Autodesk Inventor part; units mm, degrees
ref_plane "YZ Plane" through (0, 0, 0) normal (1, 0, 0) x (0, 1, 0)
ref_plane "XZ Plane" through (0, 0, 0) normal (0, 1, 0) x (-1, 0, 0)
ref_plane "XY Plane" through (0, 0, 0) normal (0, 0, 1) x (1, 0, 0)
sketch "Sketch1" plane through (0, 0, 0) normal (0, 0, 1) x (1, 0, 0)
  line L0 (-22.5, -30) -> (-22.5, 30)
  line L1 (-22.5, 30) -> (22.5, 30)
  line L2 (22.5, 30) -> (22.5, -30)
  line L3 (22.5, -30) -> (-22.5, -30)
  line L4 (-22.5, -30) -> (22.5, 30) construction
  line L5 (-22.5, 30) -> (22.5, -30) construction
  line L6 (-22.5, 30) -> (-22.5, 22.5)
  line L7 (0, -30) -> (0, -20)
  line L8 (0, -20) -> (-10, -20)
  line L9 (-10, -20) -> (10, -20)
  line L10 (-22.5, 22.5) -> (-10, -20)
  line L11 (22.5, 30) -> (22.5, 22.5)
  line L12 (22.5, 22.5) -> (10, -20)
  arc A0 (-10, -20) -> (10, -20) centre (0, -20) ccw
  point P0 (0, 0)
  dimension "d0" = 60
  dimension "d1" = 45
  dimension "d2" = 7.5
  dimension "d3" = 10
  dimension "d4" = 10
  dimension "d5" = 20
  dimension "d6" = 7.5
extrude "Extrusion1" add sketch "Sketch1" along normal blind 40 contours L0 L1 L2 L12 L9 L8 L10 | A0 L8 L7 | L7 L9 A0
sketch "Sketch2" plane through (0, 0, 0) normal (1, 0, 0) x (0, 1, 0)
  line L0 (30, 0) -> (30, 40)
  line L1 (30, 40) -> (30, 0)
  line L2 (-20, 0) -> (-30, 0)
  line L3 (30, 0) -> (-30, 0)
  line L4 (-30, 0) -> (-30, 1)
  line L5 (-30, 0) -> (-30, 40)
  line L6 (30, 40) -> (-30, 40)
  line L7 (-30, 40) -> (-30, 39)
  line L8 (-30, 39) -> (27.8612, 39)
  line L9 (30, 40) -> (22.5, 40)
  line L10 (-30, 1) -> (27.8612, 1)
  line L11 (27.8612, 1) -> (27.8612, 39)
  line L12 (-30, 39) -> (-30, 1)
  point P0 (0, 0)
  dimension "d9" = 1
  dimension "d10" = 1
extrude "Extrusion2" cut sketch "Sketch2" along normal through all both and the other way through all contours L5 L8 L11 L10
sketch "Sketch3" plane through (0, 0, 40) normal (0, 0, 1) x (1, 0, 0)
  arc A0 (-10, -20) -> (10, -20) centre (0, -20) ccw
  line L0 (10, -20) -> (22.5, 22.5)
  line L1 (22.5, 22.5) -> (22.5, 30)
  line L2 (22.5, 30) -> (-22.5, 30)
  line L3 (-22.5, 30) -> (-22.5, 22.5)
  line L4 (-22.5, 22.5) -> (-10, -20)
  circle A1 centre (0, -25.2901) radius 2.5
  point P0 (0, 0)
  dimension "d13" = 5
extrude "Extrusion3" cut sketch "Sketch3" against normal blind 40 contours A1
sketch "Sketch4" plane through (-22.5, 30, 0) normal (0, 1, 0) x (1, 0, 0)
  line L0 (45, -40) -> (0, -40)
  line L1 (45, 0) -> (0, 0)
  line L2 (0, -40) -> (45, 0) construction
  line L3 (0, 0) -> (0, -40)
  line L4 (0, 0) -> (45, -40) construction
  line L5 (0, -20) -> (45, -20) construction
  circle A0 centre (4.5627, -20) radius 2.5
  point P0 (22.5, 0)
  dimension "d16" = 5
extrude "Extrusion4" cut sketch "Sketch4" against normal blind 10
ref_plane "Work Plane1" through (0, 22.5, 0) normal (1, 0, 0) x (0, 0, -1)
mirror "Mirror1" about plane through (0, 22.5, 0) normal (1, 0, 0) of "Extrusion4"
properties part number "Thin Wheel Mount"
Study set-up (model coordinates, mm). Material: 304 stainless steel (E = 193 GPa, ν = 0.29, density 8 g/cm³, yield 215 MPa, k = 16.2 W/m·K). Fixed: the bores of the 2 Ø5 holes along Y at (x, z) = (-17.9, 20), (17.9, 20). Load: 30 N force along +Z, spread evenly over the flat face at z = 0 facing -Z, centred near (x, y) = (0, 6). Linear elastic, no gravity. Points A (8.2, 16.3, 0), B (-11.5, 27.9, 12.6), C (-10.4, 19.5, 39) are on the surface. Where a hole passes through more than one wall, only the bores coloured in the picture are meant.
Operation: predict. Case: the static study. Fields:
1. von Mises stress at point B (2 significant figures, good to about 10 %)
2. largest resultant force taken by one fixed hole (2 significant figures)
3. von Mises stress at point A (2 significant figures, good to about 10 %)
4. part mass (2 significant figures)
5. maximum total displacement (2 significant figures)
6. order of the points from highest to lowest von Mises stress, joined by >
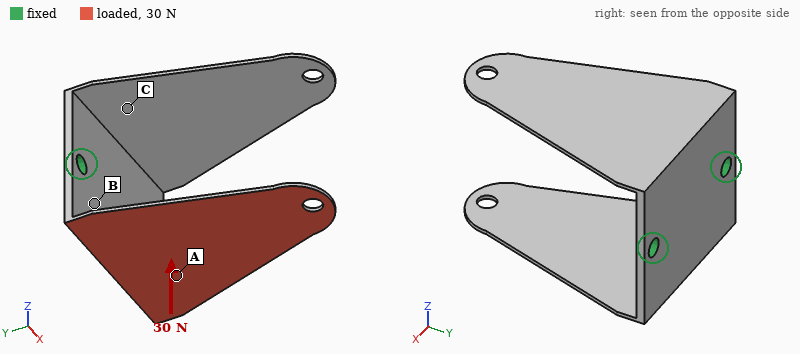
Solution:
18 MPa
16 N
50 MPa
58 g
0.86 mm
A > B > C
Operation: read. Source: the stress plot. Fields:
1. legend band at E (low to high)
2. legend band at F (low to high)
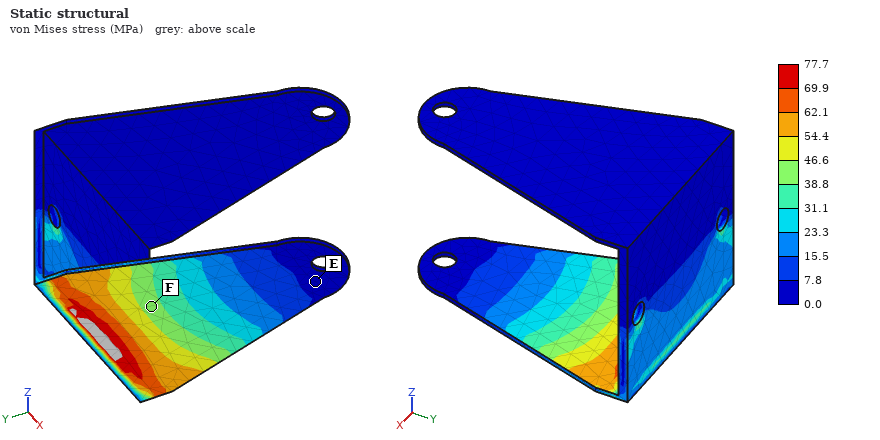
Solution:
0.0 to 7.8 MPa
38.8 to 46.6 MPa
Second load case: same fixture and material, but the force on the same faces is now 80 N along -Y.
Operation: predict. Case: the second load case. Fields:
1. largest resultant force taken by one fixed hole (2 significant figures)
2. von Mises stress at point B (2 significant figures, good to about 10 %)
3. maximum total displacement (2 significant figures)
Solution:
40 N
27 MPa
0.19 mm
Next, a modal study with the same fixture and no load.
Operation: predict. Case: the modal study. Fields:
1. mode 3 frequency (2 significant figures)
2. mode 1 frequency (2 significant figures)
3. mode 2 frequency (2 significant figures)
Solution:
1400 Hz
330 Hz
330 Hz
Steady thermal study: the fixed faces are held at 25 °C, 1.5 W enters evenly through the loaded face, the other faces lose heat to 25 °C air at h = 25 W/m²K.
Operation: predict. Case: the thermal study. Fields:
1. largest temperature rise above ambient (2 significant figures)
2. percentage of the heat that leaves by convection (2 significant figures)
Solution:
23 K
72 %
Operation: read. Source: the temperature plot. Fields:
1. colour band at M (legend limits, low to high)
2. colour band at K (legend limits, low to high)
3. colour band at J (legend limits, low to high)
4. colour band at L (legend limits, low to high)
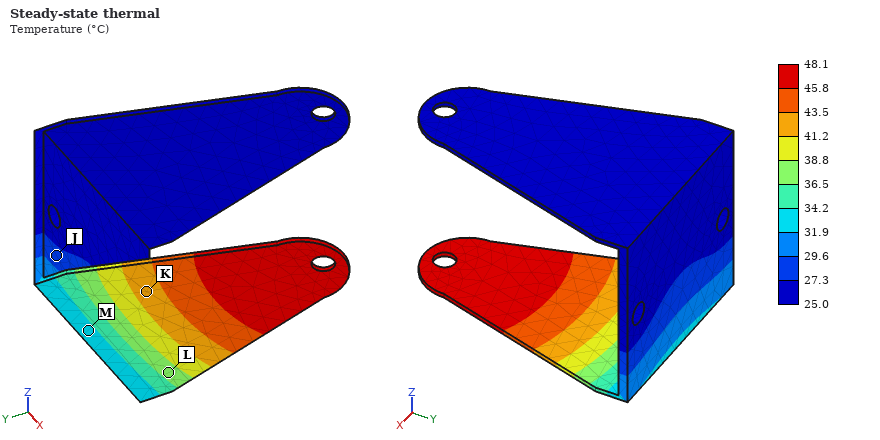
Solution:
31.9 to 34.2 °C
41.2 to 43.5 °C
27.3 to 29.6 °C
36.5 to 38.8 °C
